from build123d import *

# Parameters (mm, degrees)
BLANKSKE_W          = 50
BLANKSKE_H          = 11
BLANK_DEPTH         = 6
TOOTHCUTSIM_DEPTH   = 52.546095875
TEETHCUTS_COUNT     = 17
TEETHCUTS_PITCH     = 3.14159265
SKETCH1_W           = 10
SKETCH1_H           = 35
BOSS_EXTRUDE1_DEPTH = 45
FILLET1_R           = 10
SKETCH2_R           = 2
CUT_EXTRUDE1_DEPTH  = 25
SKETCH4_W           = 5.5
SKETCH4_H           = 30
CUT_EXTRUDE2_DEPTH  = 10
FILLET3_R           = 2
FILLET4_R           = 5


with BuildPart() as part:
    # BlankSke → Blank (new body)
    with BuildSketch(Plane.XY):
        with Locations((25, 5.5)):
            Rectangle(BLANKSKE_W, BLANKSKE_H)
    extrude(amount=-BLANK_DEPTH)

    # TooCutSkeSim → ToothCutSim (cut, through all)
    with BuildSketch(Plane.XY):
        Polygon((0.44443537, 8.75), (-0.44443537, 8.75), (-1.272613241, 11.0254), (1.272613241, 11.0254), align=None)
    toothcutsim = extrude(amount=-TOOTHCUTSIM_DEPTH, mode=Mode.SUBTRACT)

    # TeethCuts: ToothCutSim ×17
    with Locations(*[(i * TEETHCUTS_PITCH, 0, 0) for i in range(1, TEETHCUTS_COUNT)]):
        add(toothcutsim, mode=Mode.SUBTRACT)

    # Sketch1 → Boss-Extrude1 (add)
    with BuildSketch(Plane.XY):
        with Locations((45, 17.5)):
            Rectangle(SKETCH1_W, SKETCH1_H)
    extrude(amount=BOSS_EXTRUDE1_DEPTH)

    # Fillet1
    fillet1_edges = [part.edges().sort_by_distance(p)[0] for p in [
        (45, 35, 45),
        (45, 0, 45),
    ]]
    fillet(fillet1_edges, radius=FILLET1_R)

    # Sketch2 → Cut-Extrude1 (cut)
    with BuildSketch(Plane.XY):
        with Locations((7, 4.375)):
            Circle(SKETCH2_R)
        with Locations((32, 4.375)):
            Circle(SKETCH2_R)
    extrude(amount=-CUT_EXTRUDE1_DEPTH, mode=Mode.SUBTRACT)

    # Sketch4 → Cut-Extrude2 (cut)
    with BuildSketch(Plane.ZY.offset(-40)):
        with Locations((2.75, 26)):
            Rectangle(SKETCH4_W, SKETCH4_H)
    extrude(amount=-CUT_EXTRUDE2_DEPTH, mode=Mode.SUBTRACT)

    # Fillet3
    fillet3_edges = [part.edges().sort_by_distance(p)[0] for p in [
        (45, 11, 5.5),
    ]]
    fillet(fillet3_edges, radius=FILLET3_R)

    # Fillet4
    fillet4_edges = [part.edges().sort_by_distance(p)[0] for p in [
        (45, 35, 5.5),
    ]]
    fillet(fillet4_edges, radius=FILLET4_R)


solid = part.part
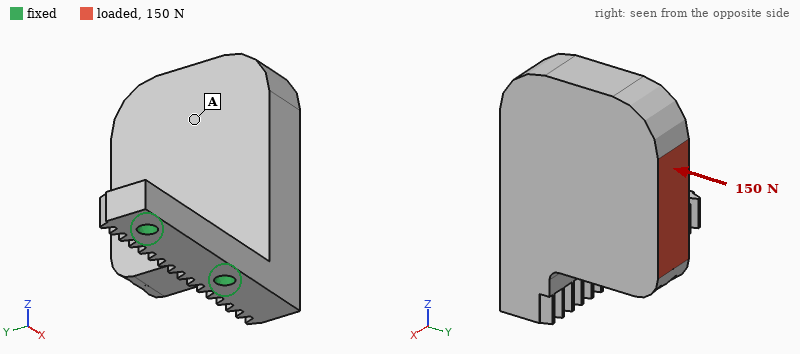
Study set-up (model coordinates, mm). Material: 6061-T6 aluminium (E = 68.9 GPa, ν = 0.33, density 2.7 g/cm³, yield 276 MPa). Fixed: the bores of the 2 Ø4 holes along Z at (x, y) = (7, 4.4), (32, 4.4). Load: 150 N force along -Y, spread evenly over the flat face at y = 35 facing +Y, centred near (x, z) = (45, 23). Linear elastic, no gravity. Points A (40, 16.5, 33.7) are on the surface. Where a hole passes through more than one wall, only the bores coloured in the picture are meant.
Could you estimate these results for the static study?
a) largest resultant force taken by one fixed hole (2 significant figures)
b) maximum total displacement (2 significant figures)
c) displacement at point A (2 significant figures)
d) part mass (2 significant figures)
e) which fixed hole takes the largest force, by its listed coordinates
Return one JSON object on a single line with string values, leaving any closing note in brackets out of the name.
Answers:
{"largest resultant force taken by one fixed hole": "170 N", "maximum total displacement": "0.20 mm", "displacement at point A": "0.14 mm", "part mass": "45 g", "which fixed hole takes the largest force, by its listed coordinates": "(32, 4.4)"}
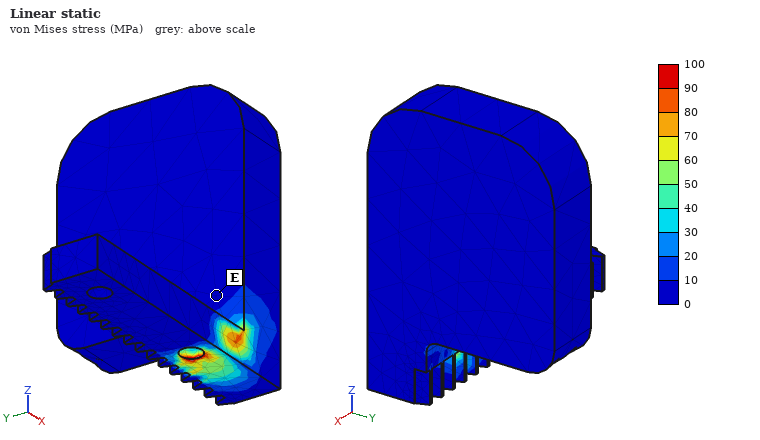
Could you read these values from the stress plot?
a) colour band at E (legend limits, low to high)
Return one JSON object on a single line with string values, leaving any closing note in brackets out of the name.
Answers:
{"colour band at E": "0 to 10 MPa"}
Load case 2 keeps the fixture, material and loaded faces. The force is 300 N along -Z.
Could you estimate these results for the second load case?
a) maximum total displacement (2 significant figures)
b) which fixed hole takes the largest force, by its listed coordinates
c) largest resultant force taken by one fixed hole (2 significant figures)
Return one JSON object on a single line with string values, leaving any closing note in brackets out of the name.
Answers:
{"maximum total displacement": "0.49 mm", "which fixed hole takes the largest force, by its listed coordinates": "(32, 4.4)", "largest resultant force taken by one fixed hole": "310 N"}
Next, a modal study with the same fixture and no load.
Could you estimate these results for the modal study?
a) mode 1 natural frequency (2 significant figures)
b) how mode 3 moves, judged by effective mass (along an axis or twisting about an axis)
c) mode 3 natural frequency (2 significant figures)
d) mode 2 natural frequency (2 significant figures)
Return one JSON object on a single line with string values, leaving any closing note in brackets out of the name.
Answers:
{"mode 1 natural frequency": "780 Hz", "how mode 3 moves, judged by effective mass": "twisting about Z", "mode 3 natural frequency": "2600 Hz", "mode 2 natural frequency": "830 Hz"}
